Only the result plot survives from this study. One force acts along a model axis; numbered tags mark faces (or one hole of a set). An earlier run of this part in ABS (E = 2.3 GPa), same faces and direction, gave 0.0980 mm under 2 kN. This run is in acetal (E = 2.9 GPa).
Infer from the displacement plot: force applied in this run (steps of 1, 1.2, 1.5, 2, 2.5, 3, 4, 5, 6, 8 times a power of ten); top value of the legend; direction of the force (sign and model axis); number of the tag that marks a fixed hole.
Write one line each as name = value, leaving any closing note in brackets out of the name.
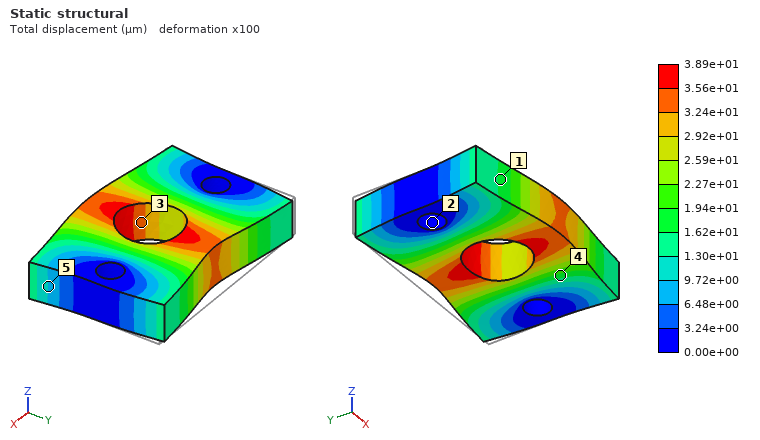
force applied in this run = 1 kN
top value of the legend = 3.89e+01 µm
direction of the force = -Y
number of the tag that marks a fixed hole = 2
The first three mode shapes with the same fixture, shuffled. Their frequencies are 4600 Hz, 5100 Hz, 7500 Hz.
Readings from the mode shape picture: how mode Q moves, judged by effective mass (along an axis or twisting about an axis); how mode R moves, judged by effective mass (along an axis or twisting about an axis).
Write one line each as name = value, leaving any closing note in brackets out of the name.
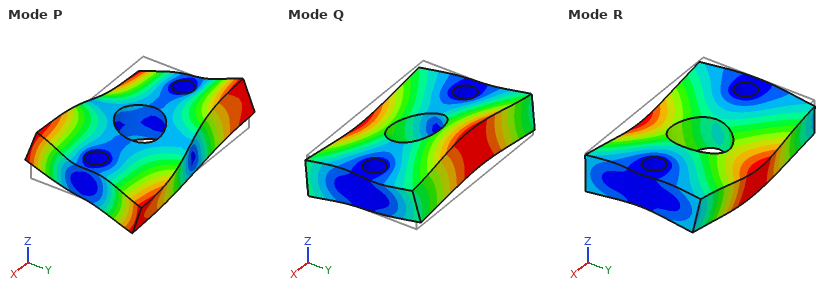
how mode Q moves, judged by effective mass = twisting about X
how mode R moves, judged by effective mass = along Z
